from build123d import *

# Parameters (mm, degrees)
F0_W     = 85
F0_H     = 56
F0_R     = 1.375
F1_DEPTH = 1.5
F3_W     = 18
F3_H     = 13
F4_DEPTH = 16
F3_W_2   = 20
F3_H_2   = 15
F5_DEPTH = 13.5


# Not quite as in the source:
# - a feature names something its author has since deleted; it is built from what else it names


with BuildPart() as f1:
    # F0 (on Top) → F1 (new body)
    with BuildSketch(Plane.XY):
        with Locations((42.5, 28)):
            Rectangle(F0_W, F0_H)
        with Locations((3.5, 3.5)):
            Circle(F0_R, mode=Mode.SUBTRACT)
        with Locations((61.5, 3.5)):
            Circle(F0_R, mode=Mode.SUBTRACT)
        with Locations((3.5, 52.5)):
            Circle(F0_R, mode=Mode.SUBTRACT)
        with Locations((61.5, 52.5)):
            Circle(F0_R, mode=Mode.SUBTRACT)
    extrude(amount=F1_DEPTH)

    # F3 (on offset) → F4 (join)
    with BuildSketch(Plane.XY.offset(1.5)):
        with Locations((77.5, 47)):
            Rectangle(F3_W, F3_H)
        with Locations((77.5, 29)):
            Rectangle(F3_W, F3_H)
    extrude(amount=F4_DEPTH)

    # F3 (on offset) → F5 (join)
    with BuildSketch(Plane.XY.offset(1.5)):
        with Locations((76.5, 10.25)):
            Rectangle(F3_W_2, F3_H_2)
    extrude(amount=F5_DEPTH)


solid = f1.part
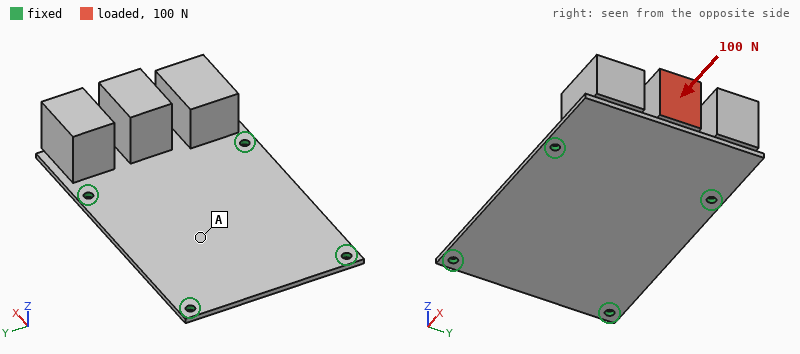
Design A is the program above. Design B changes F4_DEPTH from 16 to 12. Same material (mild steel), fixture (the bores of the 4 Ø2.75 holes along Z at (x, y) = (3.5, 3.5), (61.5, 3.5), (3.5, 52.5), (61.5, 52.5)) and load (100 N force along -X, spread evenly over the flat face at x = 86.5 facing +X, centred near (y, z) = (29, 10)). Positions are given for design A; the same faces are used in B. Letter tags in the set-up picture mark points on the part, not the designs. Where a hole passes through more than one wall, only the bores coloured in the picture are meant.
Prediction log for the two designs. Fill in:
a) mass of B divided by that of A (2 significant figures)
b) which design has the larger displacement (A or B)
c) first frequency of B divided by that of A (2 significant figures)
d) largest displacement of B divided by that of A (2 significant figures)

0.90
A
1.1
0.72
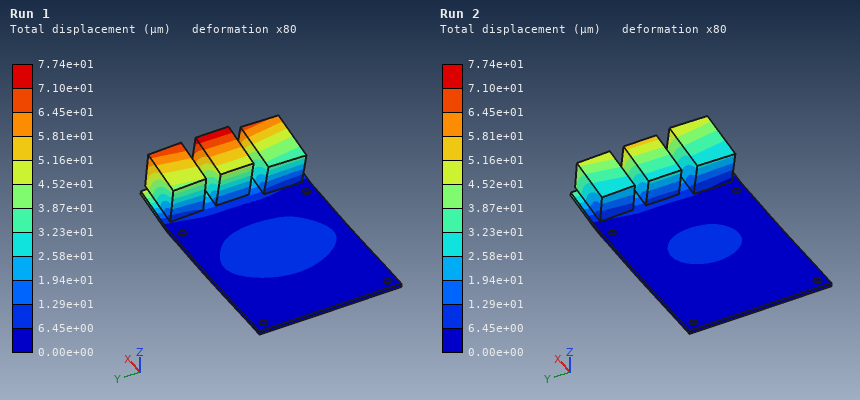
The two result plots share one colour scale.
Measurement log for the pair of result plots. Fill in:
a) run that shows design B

Run 2
